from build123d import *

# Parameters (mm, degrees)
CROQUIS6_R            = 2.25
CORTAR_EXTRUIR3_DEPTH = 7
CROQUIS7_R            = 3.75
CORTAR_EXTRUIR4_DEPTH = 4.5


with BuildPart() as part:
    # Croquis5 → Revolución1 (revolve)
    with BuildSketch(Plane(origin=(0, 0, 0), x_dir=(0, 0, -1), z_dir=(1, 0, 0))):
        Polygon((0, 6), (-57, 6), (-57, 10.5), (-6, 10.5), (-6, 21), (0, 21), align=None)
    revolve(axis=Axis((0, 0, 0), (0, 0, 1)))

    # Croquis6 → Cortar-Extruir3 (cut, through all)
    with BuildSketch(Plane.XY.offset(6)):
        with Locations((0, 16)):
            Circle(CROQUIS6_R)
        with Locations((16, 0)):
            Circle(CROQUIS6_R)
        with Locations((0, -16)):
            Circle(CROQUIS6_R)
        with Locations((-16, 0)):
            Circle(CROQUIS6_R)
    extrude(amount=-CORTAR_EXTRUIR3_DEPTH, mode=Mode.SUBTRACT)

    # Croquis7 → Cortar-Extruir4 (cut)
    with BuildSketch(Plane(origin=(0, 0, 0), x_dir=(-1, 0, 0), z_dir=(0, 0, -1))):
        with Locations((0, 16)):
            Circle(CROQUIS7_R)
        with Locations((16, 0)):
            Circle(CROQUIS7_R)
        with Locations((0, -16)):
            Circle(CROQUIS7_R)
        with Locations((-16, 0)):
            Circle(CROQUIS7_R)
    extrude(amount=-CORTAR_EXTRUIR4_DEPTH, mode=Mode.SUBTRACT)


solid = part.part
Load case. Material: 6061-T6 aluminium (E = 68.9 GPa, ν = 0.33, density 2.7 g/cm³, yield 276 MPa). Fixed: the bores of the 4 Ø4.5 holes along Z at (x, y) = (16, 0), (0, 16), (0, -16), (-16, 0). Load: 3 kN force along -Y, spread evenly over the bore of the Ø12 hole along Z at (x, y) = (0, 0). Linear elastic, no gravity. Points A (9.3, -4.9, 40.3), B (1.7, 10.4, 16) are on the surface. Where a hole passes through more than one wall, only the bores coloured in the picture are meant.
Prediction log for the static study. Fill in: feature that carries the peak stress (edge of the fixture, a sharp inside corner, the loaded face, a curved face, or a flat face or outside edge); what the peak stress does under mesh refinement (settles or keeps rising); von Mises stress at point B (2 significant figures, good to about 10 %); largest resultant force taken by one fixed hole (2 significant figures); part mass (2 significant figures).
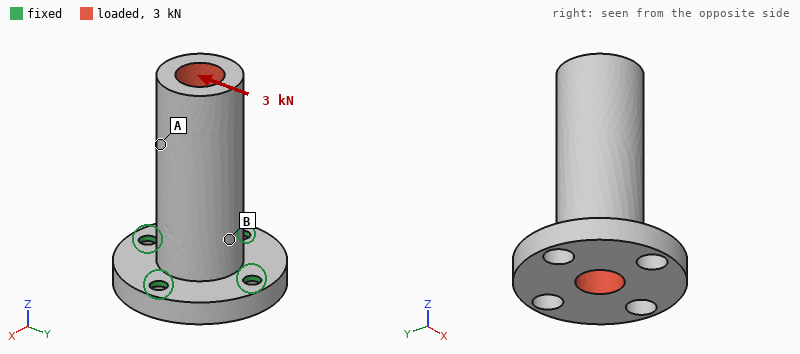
edge of the fixture
keeps rising
50 MPa
2.2 kN
50 g
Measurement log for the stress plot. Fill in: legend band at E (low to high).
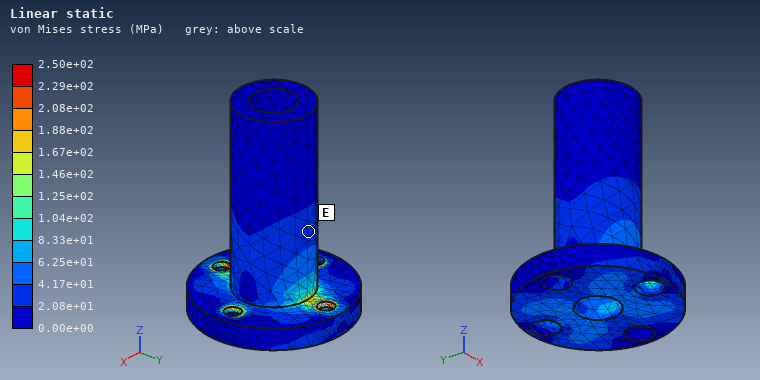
2.08e+01 to 4.17e+01 MPa
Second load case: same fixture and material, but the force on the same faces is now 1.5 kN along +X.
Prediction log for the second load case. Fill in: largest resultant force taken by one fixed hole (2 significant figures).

1.1 kN
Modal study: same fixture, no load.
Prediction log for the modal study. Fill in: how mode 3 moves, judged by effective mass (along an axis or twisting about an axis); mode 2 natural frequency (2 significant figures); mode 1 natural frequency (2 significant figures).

along Z
3700 Hz
3700 Hz
